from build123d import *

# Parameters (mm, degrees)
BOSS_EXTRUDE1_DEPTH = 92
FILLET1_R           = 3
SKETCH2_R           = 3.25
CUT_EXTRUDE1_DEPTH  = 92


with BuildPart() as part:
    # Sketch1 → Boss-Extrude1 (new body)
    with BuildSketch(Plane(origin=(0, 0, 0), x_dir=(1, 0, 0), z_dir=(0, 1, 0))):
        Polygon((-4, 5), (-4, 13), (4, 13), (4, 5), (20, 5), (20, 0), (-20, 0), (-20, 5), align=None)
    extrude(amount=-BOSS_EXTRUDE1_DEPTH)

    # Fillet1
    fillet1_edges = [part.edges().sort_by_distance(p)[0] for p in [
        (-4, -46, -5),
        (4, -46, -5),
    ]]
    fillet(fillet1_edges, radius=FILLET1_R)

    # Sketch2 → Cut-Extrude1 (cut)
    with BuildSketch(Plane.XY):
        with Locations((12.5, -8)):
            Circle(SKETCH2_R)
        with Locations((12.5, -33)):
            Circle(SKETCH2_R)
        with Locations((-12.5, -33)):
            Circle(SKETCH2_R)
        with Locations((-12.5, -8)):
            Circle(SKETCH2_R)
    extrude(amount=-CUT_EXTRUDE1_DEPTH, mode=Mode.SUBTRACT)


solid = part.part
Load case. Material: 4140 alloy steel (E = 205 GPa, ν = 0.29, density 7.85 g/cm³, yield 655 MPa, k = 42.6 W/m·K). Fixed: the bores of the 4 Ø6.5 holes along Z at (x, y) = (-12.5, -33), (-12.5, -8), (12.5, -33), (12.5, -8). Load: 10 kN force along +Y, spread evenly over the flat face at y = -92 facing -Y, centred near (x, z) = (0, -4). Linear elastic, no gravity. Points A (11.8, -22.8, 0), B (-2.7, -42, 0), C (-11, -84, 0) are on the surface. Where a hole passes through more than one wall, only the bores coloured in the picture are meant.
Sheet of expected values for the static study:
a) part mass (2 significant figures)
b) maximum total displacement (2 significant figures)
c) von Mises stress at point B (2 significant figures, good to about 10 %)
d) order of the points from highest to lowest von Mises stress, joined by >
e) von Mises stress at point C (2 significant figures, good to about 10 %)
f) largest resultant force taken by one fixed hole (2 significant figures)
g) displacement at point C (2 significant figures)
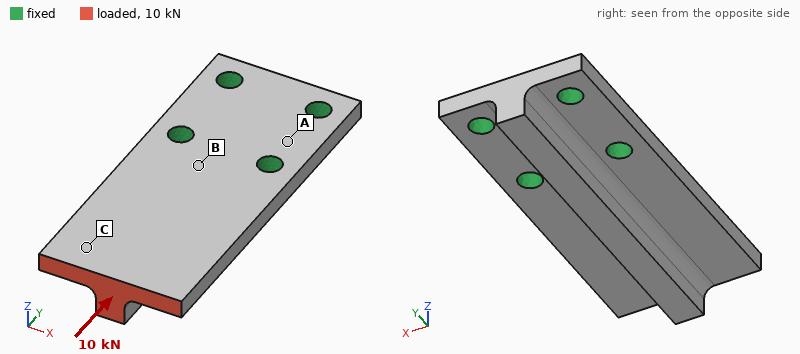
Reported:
190 g
22 µm
24 MPa
C > B > A
37 MPa
4.2 kN
16 µm
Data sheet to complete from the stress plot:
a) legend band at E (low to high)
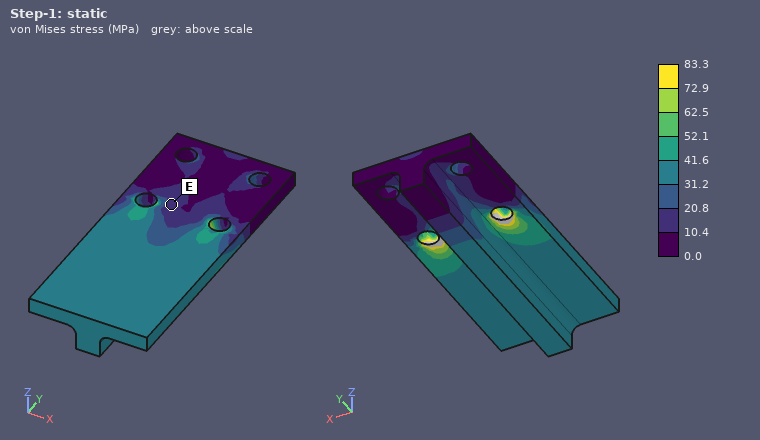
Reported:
10.4 to 20.8 MPa
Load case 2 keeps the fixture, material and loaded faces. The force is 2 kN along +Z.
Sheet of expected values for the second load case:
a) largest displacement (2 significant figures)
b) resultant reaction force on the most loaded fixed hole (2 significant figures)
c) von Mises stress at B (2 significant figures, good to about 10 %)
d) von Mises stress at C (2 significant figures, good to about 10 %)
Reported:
0.34 mm
3.5 kN
180 MPa
34 MPa
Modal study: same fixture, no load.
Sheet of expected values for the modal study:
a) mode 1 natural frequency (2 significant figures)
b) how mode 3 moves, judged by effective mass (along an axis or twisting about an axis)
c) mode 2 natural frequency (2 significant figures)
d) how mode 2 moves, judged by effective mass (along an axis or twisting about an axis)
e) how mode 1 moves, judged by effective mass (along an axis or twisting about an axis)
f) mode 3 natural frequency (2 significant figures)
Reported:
2100 Hz
along X
5100 Hz
twisting about Y
along Z
6700 Hz
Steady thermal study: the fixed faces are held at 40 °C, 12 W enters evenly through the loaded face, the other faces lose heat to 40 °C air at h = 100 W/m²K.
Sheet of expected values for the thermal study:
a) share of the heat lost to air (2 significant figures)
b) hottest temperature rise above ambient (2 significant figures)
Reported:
69 %
34 K
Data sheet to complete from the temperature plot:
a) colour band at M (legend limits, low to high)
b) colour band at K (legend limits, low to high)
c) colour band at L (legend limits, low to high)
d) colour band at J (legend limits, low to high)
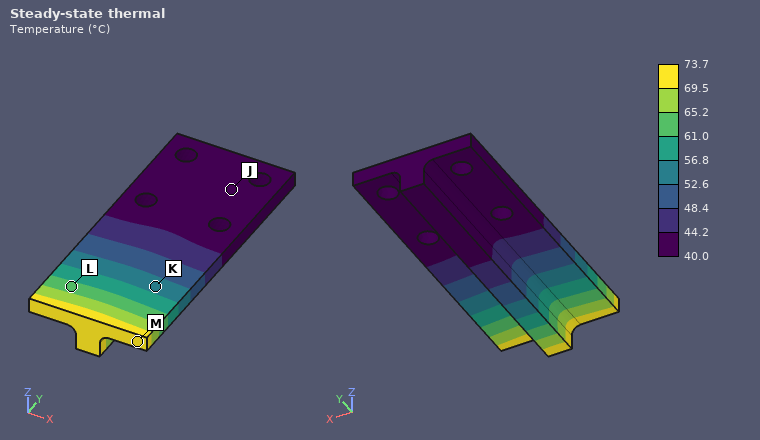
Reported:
69.5 to 73.7 °C
52.6 to 56.8 °C
61.0 to 65.2 °C
40.0 to 44.2 °C
